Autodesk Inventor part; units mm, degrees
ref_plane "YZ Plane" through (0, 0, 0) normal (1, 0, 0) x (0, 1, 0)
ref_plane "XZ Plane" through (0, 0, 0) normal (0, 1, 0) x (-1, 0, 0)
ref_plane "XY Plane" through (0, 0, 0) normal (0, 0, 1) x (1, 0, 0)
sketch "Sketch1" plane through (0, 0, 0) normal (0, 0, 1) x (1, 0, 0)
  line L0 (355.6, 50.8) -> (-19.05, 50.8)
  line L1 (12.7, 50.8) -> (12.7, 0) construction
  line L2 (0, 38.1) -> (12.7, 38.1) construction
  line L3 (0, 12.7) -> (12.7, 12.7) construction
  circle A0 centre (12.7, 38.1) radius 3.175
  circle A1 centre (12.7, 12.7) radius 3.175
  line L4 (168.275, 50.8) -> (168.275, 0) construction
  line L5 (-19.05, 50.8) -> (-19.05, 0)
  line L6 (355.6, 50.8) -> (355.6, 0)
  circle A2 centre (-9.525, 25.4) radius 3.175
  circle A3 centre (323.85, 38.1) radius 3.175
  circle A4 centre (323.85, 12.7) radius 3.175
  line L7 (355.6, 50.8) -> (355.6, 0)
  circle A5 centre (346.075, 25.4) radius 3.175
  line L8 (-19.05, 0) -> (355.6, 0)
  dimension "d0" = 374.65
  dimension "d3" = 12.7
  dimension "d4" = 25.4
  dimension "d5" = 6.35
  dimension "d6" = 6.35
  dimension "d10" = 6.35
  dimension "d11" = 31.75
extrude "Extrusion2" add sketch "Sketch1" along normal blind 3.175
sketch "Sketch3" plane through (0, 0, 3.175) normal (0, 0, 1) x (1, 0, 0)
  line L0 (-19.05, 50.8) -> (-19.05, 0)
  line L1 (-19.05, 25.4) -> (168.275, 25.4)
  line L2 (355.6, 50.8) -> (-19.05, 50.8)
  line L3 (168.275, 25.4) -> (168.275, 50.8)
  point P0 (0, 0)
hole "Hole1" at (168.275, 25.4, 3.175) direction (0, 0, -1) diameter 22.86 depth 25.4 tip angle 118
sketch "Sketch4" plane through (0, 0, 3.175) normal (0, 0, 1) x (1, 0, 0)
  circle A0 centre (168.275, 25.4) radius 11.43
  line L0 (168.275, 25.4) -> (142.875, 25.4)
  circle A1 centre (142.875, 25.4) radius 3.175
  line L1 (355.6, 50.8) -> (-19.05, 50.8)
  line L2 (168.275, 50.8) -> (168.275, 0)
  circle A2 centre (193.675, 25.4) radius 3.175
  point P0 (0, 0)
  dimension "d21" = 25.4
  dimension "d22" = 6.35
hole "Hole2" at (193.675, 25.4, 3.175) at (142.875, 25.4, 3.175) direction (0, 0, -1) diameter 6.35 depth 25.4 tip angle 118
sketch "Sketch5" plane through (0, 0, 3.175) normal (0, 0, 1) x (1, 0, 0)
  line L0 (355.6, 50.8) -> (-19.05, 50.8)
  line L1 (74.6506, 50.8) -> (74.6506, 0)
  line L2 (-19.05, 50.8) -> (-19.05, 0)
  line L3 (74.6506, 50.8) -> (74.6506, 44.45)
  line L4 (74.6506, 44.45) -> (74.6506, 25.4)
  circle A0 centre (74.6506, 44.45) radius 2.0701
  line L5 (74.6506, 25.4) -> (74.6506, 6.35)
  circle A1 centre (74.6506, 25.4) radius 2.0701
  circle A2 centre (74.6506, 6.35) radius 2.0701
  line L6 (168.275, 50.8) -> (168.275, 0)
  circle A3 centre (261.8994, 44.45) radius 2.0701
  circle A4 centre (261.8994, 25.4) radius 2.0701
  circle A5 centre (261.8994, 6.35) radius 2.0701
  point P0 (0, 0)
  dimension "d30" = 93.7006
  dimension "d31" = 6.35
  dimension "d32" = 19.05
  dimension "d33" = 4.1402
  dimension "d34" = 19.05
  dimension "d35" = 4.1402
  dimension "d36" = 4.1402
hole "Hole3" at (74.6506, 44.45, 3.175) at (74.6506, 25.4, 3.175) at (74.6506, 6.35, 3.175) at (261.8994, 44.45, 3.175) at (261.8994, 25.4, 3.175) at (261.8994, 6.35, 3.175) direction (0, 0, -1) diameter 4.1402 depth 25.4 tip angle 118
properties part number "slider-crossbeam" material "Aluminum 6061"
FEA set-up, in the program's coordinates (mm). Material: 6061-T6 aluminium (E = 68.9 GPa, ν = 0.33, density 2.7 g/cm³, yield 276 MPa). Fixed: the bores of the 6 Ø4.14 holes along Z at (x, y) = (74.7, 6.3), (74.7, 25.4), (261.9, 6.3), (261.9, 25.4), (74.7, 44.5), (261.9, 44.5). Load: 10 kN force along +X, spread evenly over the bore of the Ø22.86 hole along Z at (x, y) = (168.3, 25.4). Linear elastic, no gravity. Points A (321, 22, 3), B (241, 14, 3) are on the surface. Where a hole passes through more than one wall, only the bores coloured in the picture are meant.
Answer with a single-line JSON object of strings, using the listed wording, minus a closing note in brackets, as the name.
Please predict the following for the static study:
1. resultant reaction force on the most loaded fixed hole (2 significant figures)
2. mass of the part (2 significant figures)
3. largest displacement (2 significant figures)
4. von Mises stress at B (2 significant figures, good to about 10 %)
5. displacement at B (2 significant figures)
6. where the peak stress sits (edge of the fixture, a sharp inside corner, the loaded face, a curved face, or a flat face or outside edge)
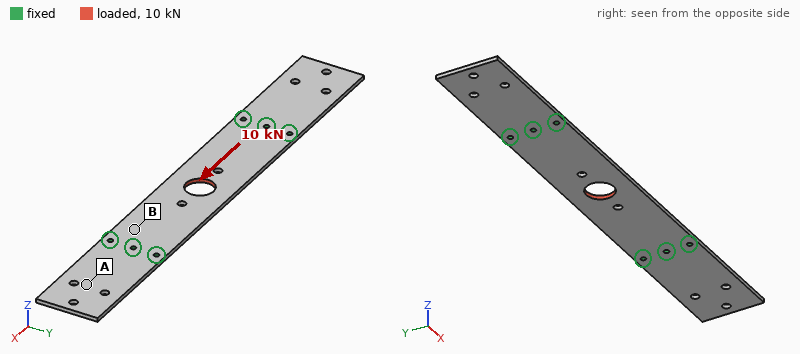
{"resultant reaction force on the most loaded fixed hole": "1.7 kN", "mass of the part": "160 g", "largest displacement": "46 µm", "von Mises stress at B": "31 MPa", "displacement at B": "10 µm", "where the peak stress sits": "a curved face"}
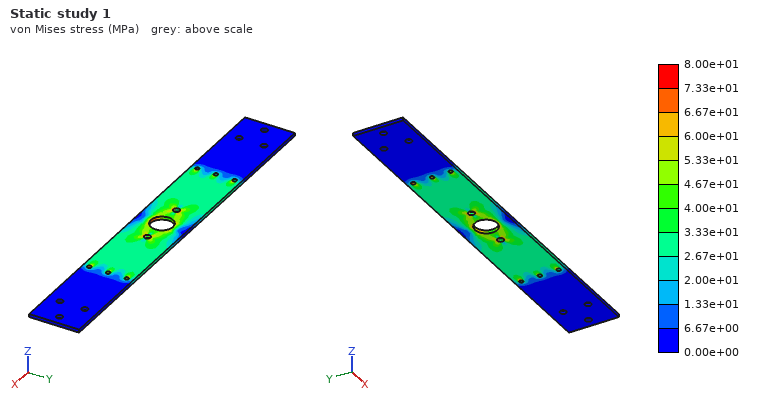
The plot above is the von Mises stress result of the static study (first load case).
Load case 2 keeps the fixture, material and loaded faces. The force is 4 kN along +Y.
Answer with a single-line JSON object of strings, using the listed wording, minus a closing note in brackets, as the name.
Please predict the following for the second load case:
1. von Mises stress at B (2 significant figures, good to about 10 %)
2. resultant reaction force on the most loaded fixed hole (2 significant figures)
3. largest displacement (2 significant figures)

{"von Mises stress at B": "31 MPa", "resultant reaction force on the most loaded fixed hole": "2.4 kN", "largest displacement": "0.11 mm"}
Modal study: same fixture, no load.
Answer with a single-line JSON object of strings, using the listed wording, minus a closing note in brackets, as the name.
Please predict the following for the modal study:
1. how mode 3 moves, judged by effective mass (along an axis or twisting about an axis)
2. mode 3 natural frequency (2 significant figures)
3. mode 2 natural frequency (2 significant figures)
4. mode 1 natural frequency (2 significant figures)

{"how mode 3 moves, judged by effective mass": "along Z", "mode 3 natural frequency": "490 Hz", "mode 2 natural frequency": "310 Hz", "mode 1 natural frequency": "310 Hz"}
